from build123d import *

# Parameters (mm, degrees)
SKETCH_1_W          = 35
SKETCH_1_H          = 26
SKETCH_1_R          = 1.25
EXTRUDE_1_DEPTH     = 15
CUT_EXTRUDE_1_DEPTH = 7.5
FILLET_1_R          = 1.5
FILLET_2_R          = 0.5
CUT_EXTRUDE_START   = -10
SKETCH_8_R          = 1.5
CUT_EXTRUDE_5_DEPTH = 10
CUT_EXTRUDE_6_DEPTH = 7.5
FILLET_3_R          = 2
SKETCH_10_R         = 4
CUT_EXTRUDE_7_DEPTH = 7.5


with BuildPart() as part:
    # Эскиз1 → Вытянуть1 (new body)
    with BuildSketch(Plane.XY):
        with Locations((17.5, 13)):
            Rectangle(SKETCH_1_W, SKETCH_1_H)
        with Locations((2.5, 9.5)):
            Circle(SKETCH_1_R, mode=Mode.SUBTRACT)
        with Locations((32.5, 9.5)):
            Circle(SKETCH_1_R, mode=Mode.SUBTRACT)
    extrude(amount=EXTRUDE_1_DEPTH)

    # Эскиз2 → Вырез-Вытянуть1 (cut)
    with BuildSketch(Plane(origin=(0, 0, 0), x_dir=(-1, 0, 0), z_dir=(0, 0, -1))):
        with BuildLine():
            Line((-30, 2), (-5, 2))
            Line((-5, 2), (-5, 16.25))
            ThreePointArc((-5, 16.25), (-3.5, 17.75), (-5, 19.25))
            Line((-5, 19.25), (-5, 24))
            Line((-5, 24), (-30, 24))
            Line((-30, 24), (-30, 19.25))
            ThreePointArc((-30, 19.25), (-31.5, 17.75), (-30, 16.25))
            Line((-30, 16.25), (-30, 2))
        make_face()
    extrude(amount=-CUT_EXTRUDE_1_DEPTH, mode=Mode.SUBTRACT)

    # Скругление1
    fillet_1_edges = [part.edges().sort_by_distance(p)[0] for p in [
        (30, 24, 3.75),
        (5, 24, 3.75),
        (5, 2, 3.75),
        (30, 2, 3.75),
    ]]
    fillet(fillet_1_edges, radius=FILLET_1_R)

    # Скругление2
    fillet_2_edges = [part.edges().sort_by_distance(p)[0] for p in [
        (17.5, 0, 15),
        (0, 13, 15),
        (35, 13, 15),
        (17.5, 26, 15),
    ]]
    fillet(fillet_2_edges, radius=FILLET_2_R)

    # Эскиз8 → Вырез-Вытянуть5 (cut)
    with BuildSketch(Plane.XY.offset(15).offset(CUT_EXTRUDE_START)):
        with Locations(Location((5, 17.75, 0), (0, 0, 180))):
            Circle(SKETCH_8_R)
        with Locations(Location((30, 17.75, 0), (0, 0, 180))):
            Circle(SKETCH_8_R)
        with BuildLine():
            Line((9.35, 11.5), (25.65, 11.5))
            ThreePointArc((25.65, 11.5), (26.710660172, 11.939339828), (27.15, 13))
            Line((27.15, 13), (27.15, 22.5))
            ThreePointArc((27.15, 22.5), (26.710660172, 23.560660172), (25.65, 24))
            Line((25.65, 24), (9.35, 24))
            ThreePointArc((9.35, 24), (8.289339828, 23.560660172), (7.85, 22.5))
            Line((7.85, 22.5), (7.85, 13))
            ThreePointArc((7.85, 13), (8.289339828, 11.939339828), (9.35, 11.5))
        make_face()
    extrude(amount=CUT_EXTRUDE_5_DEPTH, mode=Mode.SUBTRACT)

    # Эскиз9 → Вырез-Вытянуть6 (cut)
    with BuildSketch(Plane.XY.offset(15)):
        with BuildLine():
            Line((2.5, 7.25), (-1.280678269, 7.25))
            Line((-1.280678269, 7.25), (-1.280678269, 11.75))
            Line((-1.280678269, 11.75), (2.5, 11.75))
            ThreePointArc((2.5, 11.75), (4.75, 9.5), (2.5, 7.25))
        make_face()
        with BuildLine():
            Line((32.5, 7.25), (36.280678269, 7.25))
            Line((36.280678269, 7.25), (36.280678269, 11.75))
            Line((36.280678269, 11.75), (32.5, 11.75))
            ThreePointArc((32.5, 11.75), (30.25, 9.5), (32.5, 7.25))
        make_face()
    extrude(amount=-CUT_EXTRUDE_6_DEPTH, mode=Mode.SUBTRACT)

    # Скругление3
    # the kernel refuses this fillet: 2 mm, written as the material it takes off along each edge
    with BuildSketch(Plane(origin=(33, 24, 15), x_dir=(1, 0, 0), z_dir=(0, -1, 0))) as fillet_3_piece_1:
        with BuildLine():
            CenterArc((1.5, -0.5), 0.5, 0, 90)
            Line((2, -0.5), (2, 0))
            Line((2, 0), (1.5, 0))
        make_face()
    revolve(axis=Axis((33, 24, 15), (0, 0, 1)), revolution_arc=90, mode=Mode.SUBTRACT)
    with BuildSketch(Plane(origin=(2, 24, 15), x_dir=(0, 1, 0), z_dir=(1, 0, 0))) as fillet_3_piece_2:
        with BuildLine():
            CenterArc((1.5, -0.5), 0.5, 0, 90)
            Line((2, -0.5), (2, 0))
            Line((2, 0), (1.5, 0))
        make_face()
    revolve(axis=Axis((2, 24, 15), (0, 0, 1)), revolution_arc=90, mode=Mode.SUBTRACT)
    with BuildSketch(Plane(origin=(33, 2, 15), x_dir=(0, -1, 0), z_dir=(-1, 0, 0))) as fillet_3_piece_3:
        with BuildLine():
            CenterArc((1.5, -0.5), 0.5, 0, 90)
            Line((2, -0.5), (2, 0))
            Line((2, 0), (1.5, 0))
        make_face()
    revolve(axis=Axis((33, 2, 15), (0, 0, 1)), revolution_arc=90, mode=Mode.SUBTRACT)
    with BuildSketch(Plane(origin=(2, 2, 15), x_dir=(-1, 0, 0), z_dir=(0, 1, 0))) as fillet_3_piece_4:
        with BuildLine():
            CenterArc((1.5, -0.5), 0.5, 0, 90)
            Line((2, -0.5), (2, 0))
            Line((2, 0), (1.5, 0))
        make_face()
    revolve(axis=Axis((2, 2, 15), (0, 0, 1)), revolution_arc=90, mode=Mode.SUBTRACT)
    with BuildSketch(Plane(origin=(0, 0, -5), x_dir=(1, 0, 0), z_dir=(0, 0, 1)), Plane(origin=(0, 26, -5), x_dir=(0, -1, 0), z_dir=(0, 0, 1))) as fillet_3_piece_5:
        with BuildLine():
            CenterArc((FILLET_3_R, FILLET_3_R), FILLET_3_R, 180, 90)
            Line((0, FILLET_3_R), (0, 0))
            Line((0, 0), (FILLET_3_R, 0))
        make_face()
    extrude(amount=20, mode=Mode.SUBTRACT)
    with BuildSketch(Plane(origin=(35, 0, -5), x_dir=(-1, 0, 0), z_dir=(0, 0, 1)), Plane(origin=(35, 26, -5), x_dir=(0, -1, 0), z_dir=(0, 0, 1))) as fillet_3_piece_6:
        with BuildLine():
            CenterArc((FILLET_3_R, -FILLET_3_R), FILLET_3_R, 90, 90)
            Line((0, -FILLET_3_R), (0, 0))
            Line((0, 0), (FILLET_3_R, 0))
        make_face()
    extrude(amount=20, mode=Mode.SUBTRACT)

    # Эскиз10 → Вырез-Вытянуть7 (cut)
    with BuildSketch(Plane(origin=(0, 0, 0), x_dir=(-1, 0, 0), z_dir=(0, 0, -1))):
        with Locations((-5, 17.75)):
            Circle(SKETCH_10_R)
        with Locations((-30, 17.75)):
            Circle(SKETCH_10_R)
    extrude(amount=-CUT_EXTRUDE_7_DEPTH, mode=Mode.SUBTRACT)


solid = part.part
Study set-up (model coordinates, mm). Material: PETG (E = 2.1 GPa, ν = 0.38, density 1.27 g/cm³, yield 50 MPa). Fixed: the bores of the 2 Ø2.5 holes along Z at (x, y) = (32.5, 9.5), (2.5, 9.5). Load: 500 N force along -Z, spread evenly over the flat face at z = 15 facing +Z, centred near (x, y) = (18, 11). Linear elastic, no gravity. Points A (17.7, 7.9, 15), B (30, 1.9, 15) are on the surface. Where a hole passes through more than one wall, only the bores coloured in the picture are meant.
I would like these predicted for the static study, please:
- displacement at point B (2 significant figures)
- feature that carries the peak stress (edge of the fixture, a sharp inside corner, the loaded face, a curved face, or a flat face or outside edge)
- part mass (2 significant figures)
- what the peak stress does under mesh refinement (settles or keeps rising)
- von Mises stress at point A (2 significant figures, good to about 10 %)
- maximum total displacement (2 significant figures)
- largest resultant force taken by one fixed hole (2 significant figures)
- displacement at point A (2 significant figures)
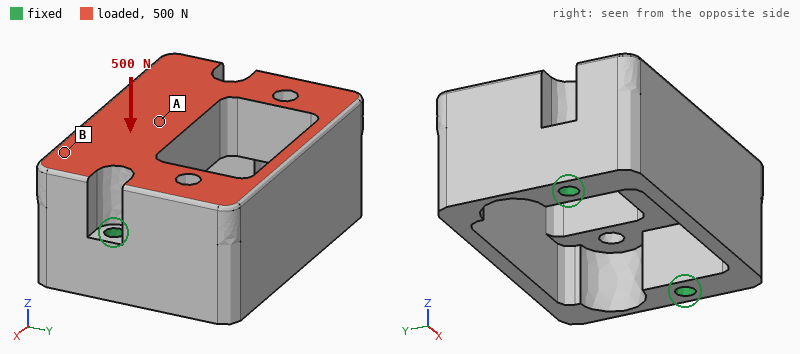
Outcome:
0.032 mm
edge of the fixture
8.7 g
keeps rising
3.9 MPa
0.18 mm
260 N
0.068 mm
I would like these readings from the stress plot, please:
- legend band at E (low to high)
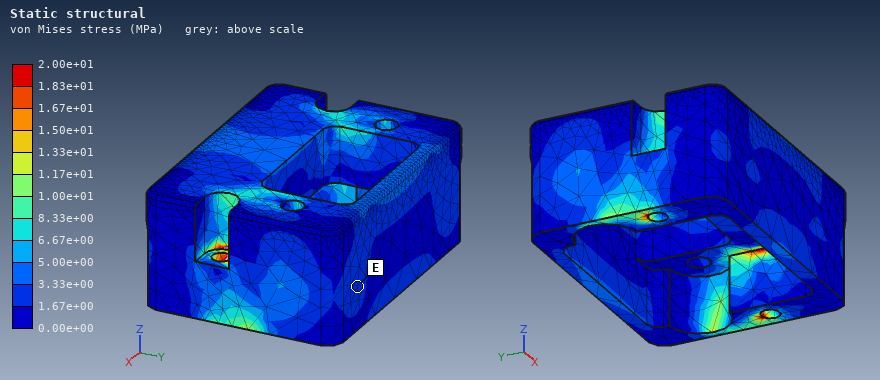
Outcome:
1.67e+00 to 3.33e+00 MPa
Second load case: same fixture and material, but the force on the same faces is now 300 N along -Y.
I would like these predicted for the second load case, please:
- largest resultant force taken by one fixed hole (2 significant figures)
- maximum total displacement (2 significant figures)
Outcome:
150 N
0.29 mm
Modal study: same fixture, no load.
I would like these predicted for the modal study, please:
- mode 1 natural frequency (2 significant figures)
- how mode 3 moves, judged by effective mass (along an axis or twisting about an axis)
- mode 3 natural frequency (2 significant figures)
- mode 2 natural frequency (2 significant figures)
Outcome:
2500 Hz
along Y
4100 Hz
2500 Hz
